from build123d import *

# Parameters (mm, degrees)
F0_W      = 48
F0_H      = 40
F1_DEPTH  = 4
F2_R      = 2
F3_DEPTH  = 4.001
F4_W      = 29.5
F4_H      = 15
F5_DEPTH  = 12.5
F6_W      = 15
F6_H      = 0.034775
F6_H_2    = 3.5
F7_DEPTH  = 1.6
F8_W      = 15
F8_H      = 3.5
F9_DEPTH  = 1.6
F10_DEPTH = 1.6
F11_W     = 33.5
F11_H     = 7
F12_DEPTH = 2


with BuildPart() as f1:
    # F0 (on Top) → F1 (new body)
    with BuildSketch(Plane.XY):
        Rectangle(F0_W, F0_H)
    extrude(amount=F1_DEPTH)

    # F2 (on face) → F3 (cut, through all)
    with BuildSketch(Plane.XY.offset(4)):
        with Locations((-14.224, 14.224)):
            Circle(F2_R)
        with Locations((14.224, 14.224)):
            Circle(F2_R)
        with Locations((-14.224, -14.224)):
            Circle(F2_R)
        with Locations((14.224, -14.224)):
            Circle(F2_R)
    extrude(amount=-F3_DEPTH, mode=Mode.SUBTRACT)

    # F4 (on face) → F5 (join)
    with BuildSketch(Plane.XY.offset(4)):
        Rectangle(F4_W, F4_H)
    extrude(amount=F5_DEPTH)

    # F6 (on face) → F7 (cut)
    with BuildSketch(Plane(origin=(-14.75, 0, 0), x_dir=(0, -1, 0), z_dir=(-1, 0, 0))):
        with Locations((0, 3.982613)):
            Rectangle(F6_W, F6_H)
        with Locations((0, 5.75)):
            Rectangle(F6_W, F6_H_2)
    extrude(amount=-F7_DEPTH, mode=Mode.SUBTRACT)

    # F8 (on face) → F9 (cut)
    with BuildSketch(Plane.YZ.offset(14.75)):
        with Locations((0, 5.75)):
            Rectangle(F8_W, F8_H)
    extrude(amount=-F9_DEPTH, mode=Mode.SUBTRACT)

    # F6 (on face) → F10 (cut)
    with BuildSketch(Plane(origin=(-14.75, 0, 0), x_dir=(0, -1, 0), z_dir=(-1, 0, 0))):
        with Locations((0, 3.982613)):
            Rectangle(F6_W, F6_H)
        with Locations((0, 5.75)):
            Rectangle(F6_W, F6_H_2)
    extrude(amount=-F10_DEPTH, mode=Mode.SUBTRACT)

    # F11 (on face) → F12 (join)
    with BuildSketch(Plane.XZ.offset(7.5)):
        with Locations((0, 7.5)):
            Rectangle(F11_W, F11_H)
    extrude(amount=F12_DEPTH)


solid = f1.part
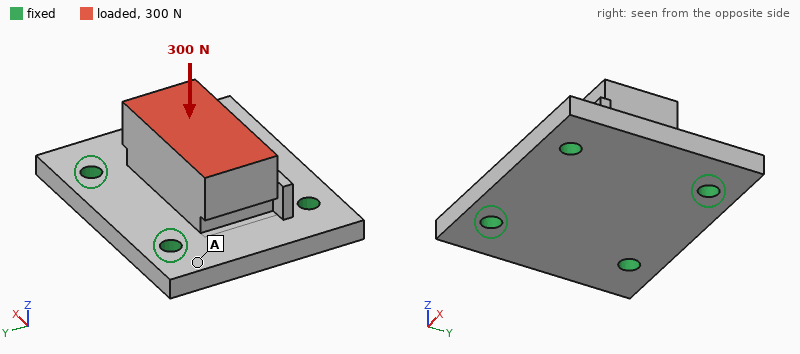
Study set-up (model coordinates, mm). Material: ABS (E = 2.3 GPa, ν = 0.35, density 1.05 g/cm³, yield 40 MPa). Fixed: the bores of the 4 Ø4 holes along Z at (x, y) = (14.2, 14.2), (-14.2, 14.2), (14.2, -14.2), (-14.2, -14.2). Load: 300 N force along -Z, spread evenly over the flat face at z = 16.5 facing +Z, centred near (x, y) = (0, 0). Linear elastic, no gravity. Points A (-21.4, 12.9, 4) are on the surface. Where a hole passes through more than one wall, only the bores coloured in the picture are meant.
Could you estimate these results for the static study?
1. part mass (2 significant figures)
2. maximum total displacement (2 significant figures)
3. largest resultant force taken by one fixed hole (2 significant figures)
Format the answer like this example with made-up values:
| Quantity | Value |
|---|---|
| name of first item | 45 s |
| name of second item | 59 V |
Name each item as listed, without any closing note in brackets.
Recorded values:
| Quantity | Value |
|---|---|
| part mass | 14 g |
| maximum total displacement | 50 µm |
| largest resultant force taken by one fixed hole | 80 N |
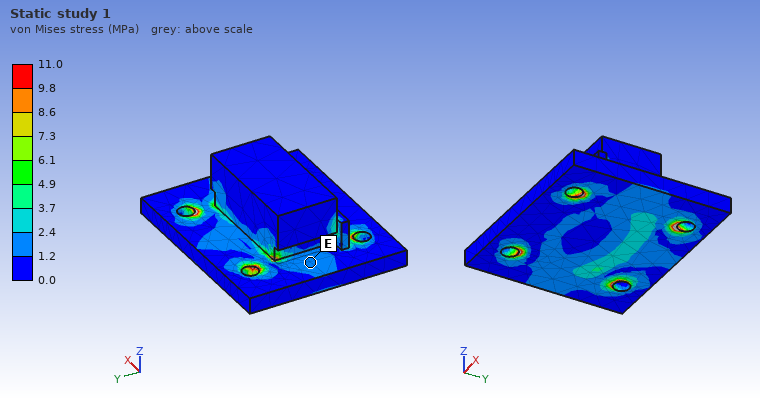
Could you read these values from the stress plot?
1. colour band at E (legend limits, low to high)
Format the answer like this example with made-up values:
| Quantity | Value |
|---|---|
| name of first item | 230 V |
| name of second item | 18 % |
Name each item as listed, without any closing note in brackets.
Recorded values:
| Quantity | Value |
|---|---|
| colour band at E | 1.2 to 2.4 MPa |
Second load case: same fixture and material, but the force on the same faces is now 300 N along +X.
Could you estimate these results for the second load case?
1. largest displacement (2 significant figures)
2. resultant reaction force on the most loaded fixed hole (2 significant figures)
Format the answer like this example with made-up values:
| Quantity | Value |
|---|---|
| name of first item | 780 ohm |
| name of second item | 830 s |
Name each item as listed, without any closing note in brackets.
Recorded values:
| Quantity | Value |
|---|---|
| largest displacement | 77 µm |
| resultant reaction force on the most loaded fixed hole | 140 N |
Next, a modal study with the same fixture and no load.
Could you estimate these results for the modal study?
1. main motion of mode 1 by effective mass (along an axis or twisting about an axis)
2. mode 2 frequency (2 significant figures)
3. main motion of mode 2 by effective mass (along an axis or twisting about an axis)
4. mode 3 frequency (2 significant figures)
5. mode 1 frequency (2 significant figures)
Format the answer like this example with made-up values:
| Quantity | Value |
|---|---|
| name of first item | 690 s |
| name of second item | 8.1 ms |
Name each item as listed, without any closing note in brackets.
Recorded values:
| Quantity | Value |
|---|---|
| main motion of mode 1 by effective mass | along Z |
| mode 2 frequency | 5200 Hz |
| main motion of mode 2 by effective mass | along X |
| mode 3 frequency | 5800 Hz |
| mode 1 frequency | 4500 Hz |
